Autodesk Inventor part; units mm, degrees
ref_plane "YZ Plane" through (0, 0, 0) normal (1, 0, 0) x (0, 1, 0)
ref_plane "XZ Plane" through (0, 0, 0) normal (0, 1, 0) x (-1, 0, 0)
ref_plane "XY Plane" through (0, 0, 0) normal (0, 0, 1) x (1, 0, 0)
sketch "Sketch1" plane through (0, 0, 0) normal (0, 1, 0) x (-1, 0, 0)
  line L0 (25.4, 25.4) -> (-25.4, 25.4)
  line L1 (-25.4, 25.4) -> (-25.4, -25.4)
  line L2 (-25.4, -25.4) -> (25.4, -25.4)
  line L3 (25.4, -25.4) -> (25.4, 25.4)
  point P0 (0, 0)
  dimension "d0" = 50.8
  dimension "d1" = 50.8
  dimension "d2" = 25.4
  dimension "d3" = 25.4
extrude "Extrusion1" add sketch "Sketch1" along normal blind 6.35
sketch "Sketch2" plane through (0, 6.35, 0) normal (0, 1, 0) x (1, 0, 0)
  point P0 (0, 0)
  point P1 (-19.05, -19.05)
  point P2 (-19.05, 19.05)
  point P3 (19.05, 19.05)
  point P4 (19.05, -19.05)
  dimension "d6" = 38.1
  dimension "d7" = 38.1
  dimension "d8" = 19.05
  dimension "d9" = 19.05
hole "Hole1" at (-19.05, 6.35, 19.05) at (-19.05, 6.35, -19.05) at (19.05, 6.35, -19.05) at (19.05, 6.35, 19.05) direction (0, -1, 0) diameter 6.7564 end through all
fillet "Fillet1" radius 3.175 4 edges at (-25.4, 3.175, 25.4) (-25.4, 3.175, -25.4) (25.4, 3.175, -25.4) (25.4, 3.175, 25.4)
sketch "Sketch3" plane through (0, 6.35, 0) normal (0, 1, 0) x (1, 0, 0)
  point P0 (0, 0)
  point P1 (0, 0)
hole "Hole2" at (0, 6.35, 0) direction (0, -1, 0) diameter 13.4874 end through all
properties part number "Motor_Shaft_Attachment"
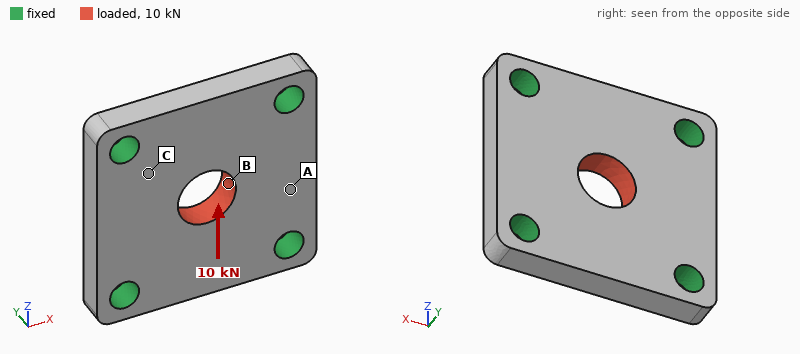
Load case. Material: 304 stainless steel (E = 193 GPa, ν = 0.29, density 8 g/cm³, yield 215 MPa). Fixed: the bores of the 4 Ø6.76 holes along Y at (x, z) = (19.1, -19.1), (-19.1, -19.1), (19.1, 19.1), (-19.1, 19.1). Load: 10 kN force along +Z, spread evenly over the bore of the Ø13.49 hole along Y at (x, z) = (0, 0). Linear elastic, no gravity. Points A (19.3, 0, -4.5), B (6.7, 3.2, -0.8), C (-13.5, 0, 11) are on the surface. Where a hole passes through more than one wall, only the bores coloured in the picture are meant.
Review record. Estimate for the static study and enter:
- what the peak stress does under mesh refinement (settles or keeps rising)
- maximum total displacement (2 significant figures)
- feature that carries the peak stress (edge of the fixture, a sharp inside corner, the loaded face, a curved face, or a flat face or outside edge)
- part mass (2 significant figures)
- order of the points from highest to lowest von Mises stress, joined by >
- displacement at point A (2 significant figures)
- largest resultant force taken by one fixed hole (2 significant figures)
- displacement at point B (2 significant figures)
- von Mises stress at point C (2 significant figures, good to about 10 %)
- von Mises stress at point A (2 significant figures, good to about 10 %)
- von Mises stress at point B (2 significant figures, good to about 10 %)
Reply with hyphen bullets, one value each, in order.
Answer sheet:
- keeps rising
- 4.5 µm
- edge of the fixture
- 120 g
- B > C > A
- 0.88 µm
- 2.8 kN
- 3.8 µm
- 33 MPa
- 11 MPa
- 65 MPa
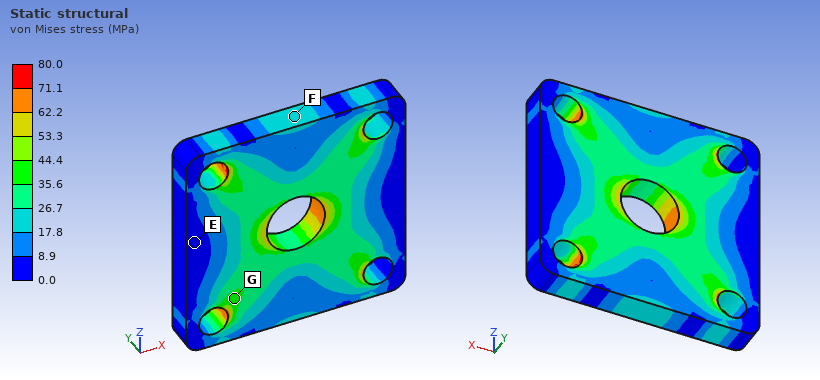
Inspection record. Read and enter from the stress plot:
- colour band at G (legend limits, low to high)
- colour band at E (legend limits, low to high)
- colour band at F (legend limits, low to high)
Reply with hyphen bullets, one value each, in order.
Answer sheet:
- 35.6 to 44.4 MPa
- 0.0 to 8.9 MPa
- 17.8 to 26.7 MPa
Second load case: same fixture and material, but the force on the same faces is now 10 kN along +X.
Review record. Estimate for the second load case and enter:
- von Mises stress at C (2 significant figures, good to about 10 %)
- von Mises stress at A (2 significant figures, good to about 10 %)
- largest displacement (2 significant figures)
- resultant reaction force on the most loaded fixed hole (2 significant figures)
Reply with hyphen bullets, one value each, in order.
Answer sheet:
- 34 MPa
- 14 MPa
- 4.5 µm
- 2.8 kN
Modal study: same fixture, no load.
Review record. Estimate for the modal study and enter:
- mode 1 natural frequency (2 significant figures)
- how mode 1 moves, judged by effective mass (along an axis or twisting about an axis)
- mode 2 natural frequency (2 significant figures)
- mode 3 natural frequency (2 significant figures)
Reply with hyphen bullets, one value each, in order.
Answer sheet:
- 17 kHz
- along Y
- 24 kHz
- 24 kHz
